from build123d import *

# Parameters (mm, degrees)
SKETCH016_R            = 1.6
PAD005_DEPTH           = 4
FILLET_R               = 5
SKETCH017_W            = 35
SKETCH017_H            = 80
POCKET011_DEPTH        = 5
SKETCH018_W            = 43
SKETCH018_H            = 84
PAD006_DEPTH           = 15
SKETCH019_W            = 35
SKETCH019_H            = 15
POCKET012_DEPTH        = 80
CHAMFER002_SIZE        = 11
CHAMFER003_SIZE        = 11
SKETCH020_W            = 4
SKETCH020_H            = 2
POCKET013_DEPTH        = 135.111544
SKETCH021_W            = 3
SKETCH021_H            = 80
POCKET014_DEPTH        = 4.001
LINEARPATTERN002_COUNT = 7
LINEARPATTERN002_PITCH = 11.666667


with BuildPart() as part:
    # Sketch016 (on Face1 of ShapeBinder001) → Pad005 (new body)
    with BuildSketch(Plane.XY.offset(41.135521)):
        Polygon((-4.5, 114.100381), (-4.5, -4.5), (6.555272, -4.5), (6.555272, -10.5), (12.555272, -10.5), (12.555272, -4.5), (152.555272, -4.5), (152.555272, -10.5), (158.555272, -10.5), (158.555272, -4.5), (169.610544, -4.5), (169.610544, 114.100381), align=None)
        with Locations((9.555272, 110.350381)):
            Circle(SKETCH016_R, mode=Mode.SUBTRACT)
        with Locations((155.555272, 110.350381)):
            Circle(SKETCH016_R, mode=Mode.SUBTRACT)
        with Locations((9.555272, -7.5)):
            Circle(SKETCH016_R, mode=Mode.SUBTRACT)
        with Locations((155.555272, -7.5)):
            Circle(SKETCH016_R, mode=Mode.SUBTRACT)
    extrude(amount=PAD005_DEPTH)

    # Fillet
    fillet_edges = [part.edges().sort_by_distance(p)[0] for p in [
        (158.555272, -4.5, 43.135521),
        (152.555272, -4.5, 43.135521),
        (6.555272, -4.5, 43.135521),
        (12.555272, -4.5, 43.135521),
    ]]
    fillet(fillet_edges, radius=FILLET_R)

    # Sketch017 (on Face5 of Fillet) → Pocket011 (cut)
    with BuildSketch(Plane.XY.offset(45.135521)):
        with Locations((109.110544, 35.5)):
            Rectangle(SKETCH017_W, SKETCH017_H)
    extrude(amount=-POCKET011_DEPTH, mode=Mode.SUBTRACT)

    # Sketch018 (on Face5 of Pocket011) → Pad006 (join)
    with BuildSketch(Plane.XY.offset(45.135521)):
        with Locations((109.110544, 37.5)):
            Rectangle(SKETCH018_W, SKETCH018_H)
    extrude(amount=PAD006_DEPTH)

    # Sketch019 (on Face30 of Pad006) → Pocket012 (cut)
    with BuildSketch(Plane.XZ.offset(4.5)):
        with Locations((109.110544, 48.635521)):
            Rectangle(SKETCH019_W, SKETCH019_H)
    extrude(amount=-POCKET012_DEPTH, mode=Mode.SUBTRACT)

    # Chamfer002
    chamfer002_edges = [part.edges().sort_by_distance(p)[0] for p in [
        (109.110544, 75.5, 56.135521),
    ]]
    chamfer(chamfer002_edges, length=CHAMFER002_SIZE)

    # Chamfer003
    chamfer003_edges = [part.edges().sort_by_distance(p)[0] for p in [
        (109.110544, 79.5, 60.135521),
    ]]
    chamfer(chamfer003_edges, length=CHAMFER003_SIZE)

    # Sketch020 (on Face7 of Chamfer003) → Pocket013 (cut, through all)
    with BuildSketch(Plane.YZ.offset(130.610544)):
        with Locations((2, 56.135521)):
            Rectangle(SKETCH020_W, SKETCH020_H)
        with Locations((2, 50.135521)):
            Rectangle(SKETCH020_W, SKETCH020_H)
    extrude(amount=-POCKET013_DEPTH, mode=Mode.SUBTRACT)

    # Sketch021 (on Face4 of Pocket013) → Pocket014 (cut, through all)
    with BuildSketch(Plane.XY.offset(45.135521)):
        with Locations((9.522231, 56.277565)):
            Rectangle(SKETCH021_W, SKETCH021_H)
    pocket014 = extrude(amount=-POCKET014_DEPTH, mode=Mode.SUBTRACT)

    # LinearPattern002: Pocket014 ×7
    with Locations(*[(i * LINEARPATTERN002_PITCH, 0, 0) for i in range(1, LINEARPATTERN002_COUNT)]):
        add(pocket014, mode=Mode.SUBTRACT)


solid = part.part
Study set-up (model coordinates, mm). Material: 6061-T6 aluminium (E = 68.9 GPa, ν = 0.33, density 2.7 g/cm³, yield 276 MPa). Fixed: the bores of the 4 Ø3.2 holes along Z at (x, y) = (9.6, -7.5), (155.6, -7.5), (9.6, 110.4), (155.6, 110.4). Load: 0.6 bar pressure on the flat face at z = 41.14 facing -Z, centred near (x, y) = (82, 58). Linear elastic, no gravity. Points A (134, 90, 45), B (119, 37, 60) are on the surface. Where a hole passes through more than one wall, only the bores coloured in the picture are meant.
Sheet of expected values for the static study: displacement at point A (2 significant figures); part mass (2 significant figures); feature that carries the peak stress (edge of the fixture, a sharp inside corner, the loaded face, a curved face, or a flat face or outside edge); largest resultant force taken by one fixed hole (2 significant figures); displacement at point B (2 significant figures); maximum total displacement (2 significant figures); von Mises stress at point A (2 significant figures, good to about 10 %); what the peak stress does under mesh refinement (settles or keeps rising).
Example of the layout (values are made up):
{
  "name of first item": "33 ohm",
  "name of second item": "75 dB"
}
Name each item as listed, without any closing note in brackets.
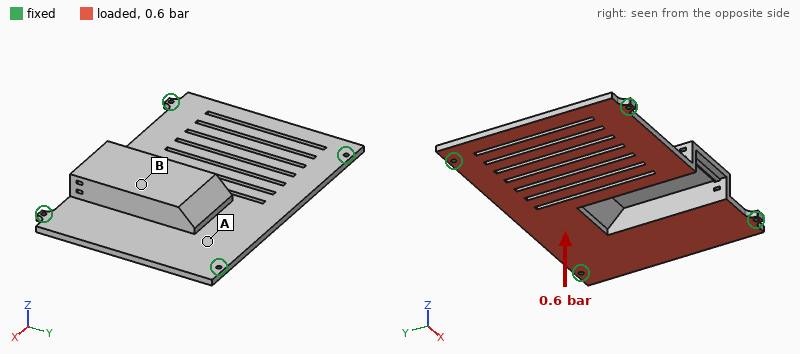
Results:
{
  "displacement at point A": "0.16 mm",
  "part mass": "240 g",
  "feature that carries the peak stress": "edge of the fixture",
  "largest resultant force taken by one fixed hole": "280 N",
  "displacement at point B": "0.26 mm",
  "maximum total displacement": "0.55 mm",
  "von Mises stress at point A": "16 MPa",
  "what the peak stress does under mesh refinement": "keeps rising"
}
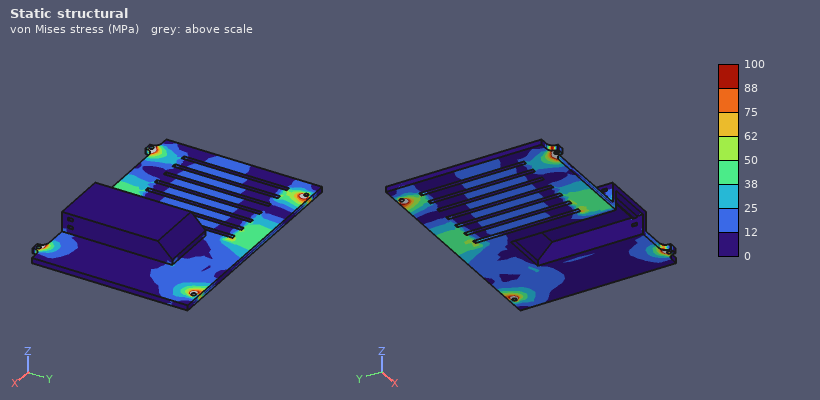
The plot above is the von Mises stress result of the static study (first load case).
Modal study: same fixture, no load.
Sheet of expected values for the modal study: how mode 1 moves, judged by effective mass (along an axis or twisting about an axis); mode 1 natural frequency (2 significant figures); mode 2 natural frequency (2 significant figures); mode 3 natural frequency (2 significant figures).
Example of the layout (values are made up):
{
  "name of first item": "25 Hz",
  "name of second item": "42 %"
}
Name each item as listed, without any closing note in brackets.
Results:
{
  "how mode 1 moves, judged by effective mass": "along Z",
  "mode 1 natural frequency": "490 Hz",
  "mode 2 natural frequency": "1200 Hz",
  "mode 3 natural frequency": "1200 Hz"
}
